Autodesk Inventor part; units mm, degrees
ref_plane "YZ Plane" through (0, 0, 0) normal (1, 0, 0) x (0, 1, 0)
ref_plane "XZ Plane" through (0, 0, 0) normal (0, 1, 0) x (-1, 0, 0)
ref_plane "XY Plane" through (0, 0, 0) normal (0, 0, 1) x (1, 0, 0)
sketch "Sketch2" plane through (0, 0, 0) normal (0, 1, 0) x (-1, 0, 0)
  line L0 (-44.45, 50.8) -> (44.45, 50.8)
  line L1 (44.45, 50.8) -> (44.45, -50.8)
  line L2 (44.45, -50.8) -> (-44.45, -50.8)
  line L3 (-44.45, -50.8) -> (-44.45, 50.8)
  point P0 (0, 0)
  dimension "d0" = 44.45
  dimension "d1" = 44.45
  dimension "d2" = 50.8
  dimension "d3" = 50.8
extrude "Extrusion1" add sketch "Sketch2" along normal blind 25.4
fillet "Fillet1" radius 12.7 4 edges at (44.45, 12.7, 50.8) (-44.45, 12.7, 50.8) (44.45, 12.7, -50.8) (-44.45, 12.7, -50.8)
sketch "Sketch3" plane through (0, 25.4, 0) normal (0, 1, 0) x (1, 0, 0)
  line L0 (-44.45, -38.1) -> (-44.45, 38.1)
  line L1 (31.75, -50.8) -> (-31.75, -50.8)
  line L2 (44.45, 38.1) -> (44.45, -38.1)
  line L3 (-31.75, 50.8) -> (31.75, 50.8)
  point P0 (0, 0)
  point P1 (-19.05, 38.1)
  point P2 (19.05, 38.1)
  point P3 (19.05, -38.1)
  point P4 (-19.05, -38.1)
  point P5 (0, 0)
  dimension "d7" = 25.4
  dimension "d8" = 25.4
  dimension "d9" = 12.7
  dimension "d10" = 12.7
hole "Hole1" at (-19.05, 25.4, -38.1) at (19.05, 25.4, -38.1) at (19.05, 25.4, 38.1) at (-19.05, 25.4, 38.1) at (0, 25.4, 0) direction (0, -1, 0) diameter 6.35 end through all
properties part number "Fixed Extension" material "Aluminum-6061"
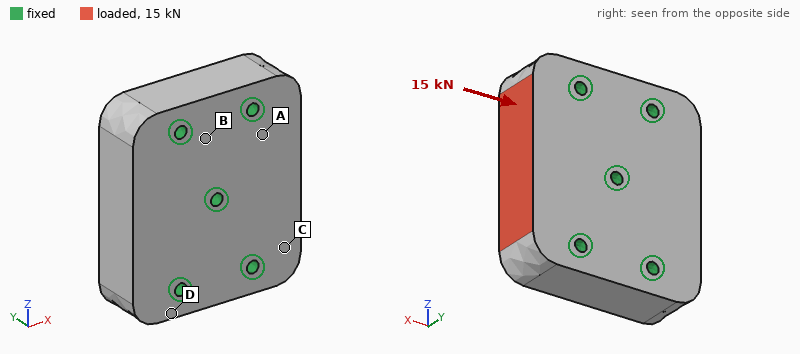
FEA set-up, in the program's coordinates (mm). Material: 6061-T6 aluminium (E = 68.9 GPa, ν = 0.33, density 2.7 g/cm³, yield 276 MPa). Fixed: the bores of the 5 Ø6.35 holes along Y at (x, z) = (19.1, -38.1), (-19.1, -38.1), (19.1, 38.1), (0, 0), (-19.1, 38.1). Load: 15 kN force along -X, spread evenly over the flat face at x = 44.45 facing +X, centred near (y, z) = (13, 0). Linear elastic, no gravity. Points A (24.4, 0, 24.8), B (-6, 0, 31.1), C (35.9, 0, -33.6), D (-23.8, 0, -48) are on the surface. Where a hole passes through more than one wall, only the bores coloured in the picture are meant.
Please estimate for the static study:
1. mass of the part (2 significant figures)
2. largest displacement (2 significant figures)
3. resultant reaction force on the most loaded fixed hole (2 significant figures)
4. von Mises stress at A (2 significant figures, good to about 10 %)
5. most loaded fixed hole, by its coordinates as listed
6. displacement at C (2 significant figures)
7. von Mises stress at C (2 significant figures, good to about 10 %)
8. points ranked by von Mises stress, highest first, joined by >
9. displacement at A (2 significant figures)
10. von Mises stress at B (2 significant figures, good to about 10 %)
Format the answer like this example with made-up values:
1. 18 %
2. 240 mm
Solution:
1. 600 g
2. 5.0 µm
3. 5.1 kN
4. 5.6 MPa
5. (0, 0)
6. 2.0 µm
7. 7.7 MPa
8. C > A > B > D
9. 2.1 µm
10. 3.3 MPa
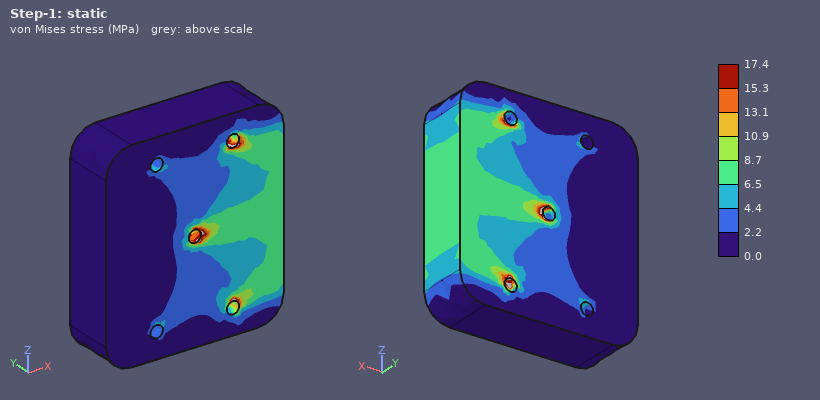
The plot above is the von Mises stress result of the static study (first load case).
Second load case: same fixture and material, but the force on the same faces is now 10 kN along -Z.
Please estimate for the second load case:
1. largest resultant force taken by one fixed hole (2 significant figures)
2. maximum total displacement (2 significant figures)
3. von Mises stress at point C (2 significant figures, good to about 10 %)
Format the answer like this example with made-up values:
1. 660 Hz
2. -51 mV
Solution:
1. 5.1 kN
2. 5.8 µm
3. 6.4 MPa
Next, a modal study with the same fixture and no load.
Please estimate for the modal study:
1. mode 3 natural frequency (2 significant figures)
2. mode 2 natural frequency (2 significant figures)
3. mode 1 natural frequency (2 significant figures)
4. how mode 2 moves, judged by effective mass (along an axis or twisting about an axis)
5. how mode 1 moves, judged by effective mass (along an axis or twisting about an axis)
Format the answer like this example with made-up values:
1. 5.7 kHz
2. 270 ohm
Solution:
1. 21 kHz
2. 13 kHz
3. 13 kHz
4. along Y
5. twisting about Z
